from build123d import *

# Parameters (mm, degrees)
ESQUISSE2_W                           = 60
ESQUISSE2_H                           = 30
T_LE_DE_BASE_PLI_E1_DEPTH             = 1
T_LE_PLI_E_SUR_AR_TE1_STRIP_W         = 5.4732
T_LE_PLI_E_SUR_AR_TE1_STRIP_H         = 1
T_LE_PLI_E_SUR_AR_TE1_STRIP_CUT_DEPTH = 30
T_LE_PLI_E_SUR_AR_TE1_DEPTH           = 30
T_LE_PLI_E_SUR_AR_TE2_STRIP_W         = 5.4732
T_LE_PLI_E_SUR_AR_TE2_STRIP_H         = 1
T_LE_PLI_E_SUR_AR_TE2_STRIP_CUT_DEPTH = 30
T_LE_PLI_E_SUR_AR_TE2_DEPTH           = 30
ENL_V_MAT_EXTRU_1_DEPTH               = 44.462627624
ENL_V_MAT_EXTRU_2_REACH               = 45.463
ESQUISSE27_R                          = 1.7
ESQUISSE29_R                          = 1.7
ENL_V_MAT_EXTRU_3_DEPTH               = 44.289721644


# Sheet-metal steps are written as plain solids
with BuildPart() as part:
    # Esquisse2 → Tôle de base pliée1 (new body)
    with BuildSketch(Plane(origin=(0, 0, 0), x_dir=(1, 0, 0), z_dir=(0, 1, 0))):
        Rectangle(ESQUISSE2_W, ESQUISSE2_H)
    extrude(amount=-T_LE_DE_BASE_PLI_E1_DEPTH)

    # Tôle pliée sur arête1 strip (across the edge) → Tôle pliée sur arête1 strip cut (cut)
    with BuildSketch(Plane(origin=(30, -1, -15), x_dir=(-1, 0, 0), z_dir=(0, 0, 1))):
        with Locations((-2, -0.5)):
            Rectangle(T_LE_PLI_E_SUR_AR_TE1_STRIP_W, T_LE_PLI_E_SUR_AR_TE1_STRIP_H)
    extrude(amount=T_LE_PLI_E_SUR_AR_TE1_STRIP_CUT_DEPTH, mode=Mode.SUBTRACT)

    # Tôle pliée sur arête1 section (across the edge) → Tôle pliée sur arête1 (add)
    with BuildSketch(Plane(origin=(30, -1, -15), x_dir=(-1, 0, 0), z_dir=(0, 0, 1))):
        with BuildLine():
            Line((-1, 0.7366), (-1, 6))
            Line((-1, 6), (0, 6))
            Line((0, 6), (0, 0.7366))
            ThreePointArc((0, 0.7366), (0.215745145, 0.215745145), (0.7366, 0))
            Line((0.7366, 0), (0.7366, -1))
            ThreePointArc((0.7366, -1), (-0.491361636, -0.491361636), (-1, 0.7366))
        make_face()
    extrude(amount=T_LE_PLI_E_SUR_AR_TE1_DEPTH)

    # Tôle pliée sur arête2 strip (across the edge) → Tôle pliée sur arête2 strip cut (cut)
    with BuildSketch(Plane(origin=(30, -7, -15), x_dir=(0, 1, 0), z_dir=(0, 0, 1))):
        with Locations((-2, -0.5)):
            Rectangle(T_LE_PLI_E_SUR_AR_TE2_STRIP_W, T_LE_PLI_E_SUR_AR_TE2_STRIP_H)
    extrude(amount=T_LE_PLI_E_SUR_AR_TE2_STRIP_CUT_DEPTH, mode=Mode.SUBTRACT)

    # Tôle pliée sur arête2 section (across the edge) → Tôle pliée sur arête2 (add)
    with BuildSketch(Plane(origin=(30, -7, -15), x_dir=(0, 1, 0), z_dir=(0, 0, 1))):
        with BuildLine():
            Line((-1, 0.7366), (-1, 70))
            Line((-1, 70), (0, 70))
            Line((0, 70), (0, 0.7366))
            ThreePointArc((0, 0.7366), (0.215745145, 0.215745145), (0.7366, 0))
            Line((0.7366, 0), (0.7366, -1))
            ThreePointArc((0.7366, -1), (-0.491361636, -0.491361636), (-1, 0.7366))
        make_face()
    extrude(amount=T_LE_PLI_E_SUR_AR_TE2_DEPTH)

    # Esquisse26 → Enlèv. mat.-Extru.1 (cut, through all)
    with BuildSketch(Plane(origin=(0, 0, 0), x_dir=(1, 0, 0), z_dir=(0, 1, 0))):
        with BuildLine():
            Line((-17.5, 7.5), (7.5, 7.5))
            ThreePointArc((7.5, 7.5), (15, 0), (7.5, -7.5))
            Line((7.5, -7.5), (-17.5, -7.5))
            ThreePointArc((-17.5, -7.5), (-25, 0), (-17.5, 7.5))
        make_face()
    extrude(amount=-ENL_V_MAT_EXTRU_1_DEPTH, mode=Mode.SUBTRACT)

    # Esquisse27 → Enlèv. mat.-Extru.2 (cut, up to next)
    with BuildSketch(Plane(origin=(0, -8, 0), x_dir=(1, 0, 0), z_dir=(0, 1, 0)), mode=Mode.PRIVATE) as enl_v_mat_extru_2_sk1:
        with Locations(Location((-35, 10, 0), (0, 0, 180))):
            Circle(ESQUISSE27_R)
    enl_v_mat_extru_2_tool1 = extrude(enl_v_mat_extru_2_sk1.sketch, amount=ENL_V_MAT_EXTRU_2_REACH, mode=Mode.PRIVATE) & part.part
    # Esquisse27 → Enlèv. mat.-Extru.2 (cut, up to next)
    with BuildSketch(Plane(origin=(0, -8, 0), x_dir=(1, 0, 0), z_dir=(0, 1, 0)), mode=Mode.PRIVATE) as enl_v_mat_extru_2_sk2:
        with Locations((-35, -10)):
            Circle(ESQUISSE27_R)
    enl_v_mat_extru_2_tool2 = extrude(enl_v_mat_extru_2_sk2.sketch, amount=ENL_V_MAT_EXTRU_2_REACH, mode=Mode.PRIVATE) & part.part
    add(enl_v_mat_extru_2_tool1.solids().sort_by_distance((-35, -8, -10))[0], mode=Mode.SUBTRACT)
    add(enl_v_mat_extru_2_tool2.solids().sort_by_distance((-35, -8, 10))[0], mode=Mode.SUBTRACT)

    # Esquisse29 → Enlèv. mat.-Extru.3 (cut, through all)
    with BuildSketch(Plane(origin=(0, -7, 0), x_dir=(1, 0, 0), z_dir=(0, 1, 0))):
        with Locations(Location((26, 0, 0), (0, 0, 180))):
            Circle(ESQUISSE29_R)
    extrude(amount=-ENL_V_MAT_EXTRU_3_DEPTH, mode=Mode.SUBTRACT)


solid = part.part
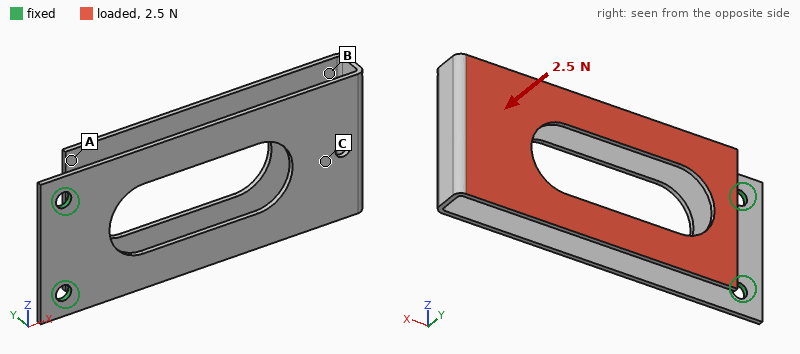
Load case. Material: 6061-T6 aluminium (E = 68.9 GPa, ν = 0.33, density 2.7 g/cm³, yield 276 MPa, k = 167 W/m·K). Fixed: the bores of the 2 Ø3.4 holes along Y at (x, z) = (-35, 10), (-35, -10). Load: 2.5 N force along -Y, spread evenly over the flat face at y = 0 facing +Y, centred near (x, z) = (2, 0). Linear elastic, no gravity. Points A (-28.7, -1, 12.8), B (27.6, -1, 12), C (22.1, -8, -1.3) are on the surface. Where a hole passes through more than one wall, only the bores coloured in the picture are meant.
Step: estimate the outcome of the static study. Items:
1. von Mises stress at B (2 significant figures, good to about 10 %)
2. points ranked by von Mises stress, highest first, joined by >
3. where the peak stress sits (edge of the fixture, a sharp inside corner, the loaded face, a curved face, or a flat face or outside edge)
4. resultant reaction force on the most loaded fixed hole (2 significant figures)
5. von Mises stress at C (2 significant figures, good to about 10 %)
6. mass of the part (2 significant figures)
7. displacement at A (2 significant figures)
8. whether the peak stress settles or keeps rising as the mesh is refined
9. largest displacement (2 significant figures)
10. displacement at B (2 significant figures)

12 MPa
B > C > A
edge of the fixture
1.3 N
7.0 MPa
8.0 g
0.82 mm
keeps rising
0.83 mm
0.63 mm
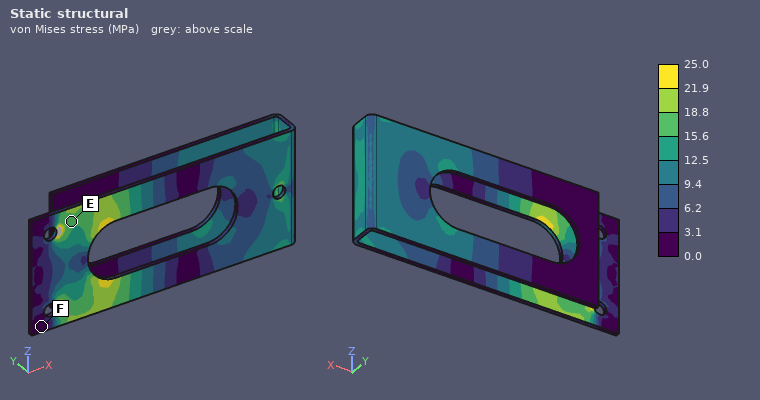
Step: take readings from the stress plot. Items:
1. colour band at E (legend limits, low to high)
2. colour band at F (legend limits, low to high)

15.6 to 18.8 MPa
0.0 to 3.1 MPa
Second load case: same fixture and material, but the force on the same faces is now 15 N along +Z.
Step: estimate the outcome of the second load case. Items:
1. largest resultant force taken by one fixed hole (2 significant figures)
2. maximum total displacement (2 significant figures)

26 N
0.89 mm
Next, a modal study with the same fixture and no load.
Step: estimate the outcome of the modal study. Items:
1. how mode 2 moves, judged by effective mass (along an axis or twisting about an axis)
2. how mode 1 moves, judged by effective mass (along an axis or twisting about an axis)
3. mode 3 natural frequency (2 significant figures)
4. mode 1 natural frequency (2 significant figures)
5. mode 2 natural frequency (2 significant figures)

along Y
along Y
310 Hz
110 Hz
160 Hz
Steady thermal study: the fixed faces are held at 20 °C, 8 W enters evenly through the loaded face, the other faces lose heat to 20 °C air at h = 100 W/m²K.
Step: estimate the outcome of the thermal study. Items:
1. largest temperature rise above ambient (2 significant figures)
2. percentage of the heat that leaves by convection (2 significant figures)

40 K
95 %
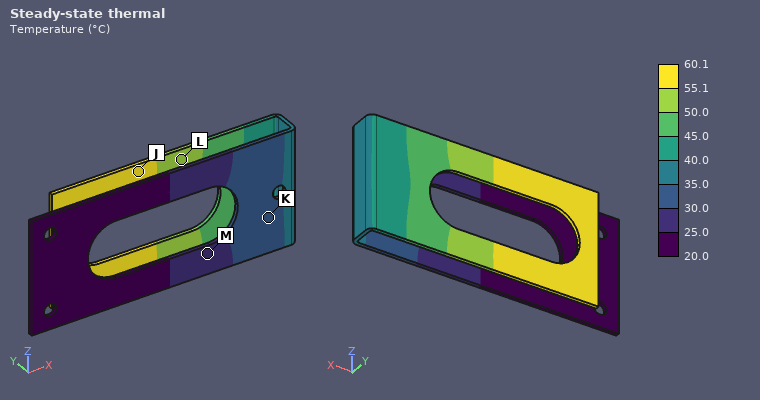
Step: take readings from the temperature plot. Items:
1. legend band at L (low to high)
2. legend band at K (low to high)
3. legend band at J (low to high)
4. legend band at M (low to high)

50.0 to 55.1 °C
30.0 to 35.0 °C
55.1 to 60.1 °C
25.0 to 30.0 °C
